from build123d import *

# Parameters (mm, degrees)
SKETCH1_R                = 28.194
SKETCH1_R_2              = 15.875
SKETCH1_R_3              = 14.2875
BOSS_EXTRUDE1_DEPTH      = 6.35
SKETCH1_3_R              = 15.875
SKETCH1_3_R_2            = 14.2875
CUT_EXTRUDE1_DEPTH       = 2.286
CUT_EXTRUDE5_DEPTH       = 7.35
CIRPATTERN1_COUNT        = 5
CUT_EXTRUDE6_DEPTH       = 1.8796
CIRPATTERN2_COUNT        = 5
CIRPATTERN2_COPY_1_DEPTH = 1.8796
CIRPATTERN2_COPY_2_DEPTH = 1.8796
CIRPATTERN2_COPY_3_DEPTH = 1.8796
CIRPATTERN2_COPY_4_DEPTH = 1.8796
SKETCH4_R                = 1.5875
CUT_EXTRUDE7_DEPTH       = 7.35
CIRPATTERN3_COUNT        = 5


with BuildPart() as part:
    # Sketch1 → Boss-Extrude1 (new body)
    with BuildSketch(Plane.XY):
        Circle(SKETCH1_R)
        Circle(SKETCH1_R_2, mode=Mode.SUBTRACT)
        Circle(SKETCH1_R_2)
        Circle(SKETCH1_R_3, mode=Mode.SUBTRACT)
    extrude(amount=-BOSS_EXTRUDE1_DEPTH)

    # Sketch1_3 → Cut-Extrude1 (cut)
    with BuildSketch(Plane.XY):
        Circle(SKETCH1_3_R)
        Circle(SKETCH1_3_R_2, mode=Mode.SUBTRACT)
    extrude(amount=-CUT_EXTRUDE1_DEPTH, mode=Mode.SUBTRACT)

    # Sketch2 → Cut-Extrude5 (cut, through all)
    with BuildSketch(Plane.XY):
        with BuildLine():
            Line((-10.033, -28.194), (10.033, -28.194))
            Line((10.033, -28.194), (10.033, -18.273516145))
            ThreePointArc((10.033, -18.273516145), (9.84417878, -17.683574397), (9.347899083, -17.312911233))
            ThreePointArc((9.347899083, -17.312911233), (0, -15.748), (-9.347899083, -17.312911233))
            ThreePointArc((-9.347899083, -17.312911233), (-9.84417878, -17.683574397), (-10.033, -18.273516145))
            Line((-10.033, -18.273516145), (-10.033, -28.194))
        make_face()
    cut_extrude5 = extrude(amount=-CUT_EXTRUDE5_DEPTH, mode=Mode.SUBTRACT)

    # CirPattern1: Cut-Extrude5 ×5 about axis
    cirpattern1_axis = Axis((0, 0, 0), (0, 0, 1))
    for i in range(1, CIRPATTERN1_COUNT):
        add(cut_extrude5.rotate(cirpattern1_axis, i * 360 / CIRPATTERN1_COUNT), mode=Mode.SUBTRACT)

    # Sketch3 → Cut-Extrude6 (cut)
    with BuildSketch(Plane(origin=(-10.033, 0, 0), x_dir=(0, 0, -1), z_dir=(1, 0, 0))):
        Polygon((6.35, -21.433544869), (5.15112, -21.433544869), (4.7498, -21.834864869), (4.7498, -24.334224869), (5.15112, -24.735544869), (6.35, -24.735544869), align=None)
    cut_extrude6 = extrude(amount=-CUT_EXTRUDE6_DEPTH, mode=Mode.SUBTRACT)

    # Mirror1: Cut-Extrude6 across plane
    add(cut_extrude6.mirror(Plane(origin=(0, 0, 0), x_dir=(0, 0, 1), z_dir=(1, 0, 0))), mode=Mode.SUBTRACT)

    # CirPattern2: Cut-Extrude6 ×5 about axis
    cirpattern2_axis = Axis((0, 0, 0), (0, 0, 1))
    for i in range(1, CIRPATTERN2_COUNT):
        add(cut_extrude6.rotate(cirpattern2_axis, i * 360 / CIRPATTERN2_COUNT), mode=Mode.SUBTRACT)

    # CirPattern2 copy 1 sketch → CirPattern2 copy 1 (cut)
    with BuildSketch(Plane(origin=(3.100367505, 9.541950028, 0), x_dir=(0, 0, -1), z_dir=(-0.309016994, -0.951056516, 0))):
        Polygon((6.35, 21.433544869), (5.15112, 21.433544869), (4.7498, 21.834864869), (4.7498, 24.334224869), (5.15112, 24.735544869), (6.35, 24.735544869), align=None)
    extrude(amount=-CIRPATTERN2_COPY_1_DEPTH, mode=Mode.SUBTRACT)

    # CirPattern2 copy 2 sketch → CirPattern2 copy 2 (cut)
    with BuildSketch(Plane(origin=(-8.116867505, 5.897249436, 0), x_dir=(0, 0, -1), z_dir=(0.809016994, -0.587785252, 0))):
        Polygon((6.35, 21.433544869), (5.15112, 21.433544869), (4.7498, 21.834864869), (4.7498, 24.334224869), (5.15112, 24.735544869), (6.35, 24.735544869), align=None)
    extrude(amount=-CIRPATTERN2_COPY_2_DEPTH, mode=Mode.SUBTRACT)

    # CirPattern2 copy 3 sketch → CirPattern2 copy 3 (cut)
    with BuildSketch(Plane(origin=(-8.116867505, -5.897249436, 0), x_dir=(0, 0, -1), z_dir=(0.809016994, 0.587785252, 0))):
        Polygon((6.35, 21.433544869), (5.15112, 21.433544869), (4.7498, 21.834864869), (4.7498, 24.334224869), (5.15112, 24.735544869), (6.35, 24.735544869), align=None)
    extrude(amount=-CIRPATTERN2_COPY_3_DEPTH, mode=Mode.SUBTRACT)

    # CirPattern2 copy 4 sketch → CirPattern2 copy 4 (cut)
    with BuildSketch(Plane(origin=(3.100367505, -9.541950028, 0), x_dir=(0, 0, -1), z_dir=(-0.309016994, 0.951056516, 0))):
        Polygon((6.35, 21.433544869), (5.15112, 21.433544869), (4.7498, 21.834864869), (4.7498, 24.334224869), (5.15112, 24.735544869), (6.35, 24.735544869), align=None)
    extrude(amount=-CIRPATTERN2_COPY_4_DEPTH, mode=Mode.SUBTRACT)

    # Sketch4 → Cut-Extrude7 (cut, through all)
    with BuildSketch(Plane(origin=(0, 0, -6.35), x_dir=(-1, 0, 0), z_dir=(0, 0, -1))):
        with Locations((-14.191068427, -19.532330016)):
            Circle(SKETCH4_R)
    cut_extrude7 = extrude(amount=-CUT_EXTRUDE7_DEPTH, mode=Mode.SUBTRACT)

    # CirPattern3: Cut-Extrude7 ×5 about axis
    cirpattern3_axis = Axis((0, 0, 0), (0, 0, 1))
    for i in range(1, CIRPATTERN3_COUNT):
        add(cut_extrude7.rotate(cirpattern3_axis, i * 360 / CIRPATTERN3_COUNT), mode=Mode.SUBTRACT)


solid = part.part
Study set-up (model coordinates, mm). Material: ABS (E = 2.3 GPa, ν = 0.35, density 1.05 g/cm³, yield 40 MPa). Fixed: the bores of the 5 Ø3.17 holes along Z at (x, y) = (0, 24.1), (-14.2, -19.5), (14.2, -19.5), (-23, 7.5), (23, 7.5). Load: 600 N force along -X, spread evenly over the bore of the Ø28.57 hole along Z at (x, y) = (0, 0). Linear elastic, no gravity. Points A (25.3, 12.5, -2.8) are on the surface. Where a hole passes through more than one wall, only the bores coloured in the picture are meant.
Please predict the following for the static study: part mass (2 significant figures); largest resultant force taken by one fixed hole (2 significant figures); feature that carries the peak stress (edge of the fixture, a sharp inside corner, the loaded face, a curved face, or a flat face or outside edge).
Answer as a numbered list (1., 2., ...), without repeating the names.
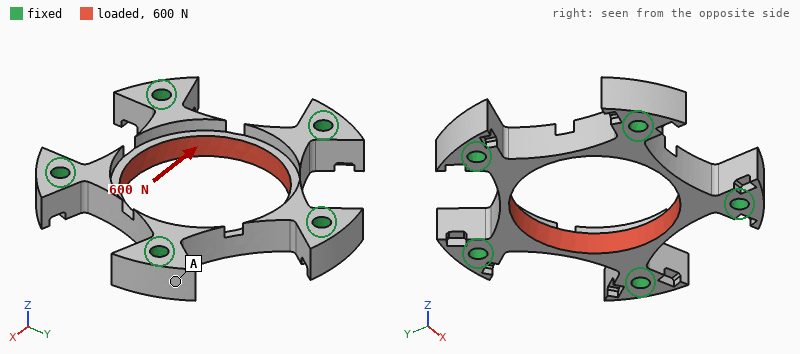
1. 4.1 g
2. 160 N
3. a curved face
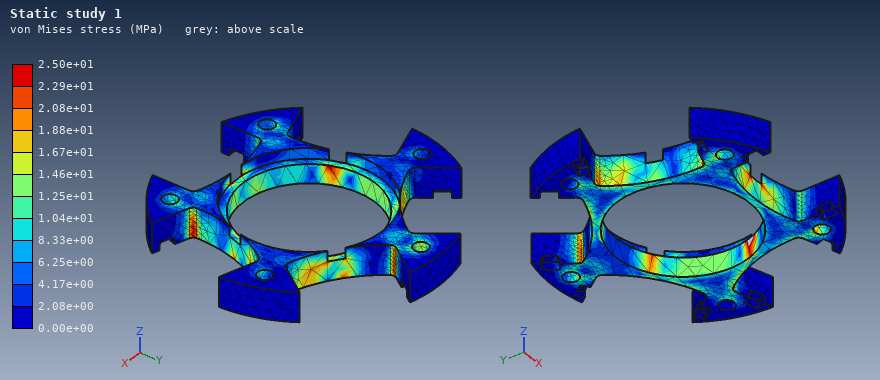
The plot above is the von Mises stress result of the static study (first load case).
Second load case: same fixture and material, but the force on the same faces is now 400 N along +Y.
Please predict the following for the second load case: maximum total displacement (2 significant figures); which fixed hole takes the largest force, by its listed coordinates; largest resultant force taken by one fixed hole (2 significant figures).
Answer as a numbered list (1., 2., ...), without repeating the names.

1. 0.13 mm
2. (0, 24.1)
3. 110 N
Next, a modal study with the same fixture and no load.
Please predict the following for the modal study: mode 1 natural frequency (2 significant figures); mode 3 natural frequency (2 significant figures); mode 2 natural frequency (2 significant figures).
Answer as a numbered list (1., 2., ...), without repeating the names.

1. 8900 Hz
2. 10 kHz
3. 8900 Hz
